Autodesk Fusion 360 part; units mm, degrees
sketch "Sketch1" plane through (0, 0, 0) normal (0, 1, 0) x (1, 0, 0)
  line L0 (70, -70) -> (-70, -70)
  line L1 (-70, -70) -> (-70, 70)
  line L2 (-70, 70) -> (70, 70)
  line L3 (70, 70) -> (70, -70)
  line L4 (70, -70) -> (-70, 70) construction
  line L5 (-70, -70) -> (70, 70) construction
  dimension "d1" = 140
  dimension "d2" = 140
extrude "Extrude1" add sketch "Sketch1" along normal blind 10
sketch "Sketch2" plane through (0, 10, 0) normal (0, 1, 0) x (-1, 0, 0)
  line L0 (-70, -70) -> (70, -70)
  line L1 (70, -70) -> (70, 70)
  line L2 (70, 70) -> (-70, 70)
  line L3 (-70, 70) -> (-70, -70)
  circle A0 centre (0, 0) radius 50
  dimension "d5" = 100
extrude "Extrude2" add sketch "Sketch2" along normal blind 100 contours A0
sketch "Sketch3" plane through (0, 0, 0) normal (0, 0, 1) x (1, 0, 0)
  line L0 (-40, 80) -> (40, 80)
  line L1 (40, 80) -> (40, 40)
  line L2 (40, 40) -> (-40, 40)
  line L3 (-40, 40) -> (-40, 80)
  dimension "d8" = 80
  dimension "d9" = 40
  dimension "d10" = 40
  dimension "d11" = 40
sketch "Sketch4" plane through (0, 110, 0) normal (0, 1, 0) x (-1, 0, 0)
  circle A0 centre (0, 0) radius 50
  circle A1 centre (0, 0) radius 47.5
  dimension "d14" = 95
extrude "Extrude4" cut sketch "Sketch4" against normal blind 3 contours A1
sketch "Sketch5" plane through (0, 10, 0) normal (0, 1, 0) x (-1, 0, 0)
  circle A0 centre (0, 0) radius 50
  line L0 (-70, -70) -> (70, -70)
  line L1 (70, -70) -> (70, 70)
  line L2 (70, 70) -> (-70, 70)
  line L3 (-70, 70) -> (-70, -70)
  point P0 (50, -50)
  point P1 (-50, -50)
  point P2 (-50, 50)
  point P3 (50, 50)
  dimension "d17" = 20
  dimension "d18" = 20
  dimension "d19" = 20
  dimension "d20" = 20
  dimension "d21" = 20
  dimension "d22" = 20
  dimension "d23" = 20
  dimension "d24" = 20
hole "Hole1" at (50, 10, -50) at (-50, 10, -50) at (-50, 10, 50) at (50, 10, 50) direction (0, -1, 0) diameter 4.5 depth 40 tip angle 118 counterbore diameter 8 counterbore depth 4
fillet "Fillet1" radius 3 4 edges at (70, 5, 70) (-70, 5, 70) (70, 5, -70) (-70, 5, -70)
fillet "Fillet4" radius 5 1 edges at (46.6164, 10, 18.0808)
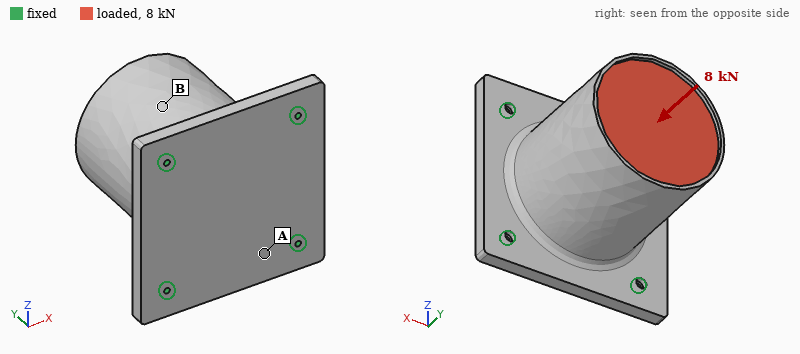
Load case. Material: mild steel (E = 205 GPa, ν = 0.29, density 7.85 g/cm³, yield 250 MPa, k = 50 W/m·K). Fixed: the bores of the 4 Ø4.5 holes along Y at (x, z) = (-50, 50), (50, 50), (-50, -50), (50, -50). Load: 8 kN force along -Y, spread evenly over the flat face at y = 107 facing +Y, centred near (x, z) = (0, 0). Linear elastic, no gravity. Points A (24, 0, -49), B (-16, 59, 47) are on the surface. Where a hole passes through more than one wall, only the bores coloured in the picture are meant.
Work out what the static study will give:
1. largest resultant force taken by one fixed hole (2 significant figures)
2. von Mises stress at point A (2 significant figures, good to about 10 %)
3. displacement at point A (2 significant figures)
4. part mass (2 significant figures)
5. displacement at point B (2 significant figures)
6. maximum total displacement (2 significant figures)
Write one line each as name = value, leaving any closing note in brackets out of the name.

largest resultant force taken by one fixed hole = 2.6 kN
von Mises stress at point A = 14 MPa
displacement at point A = 7.8 µm
part mass = 7.5 kg
displacement at point B = 9.1 µm
maximum total displacement = 9.3 µm
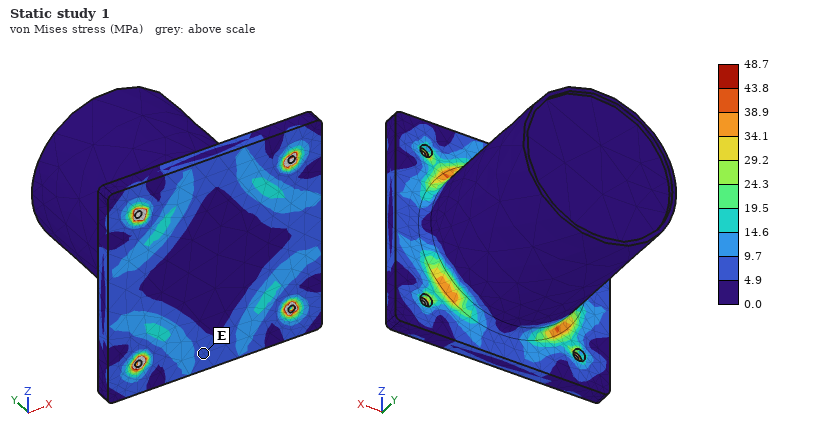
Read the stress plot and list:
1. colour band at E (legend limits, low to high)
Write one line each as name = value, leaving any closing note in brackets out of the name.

colour band at E = 4.9 to 9.7 MPa
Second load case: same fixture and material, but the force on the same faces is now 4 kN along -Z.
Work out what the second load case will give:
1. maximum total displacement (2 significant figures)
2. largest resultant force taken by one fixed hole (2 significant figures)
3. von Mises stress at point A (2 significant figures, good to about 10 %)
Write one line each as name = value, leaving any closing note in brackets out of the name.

maximum total displacement = 26 µm
largest resultant force taken by one fixed hole = 2.7 kN
von Mises stress at point A = 17 MPa
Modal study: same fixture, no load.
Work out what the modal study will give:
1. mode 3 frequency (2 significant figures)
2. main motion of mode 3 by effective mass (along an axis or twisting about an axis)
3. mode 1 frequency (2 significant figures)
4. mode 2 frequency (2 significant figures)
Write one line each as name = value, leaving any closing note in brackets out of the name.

mode 3 frequency = 1800 Hz
main motion of mode 3 by effective mass = along Y
mode 1 frequency = 1300 Hz
mode 2 frequency = 1300 Hz
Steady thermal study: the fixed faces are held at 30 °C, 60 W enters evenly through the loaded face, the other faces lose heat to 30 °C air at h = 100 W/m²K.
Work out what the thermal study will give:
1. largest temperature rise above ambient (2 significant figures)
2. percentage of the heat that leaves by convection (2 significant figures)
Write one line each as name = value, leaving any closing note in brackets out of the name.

largest temperature rise above ambient = 17 K
percentage of the heat that leaves by convection = 80 %
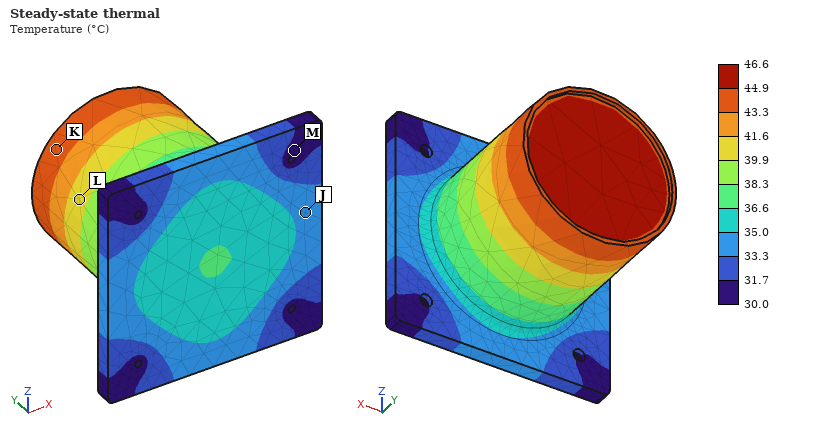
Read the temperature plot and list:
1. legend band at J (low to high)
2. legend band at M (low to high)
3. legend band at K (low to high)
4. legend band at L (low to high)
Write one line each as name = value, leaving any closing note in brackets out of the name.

legend band at J = 33.3 to 35.0 °C
legend band at M = 30.0 to 31.7 °C
legend band at K = 43.3 to 44.9 °C
legend band at L = 39.9 to 41.6 °C
